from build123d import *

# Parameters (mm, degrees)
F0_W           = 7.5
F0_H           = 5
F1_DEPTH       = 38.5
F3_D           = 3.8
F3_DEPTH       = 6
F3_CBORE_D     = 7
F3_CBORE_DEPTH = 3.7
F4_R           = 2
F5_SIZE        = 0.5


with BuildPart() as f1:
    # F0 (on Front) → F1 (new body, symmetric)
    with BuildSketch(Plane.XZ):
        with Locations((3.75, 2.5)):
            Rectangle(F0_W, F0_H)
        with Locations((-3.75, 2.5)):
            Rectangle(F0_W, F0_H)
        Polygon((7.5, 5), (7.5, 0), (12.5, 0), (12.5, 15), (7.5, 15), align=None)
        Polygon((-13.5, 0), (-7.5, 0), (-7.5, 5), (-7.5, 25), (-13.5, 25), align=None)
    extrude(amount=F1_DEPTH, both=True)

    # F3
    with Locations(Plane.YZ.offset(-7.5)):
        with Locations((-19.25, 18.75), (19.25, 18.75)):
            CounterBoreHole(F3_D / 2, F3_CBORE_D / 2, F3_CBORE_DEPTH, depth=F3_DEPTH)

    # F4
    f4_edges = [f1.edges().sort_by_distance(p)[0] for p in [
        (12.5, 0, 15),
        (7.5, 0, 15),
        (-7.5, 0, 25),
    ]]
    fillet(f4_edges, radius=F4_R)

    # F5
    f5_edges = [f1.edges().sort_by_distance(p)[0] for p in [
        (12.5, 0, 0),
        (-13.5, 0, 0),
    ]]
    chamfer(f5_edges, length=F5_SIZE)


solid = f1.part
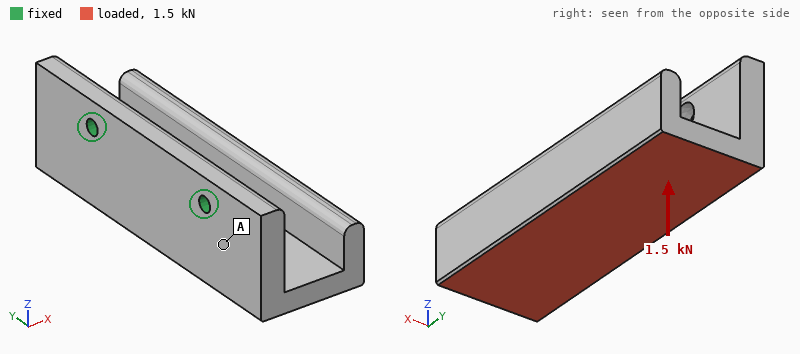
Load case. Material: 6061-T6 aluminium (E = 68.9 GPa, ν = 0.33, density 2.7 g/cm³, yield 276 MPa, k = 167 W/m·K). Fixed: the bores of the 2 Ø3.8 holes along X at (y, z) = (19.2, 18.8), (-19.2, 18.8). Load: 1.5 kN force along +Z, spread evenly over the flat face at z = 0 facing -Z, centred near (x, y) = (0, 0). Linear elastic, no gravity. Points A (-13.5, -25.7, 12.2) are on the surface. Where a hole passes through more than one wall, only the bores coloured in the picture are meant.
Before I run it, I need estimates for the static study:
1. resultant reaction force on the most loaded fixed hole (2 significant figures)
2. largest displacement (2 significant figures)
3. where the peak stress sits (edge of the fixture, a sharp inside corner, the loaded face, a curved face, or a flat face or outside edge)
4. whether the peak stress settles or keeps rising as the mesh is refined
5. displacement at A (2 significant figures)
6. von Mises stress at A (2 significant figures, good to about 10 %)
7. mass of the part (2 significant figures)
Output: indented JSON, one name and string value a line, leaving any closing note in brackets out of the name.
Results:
{
  "resultant reaction force on the most loaded fixed hole": "750 N",
  "largest displacement": "0.29 mm",
  "where the peak stress sits": "edge of the fixture",
  "whether the peak stress settles or keeps rising as the mesh is refined": "keeps rising",
  "displacement at A": "0.044 mm",
  "von Mises stress at A": "36 MPa",
  "mass of the part": "61 g"
}
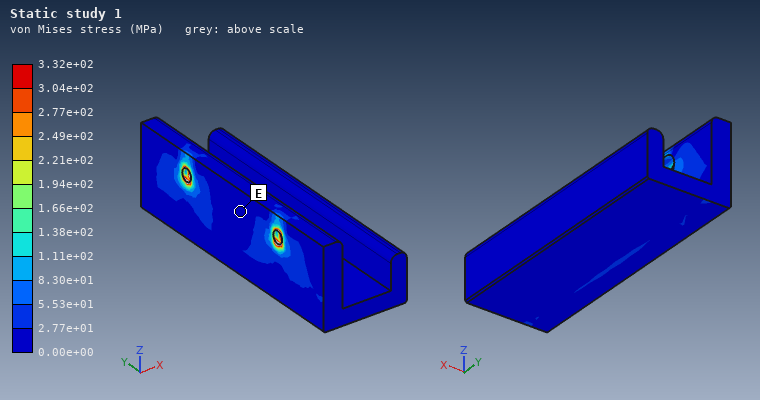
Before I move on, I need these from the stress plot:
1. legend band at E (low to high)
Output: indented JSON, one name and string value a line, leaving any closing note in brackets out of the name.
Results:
{
  "legend band at E": "0.00e+00 to 2.77e+01 MPa"
}
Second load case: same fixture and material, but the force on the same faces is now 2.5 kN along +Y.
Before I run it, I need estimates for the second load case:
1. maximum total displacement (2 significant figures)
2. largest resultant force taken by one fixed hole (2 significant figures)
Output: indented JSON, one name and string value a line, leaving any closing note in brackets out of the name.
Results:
{
  "maximum total displacement": "72 µm",
  "largest resultant force taken by one fixed hole": "1.9 kN"
}
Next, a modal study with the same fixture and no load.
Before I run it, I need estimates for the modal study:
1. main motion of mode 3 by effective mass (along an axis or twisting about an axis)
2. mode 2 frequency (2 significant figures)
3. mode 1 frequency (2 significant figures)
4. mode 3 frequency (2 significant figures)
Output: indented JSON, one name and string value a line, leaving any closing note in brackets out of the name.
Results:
{
  "main motion of mode 3 by effective mass": "along X",
  "mode 2 frequency": "3100 Hz",
  "mode 1 frequency": "1600 Hz",
  "mode 3 frequency": "5500 Hz"
}
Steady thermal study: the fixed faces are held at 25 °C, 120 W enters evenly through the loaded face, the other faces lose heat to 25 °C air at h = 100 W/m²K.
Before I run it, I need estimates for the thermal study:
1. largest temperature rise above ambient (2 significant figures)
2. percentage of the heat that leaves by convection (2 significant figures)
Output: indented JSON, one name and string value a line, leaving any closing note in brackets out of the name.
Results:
{
  "largest temperature rise above ambient": "53 K",
  "percentage of the heat that leaves by convection": "25 %"
}
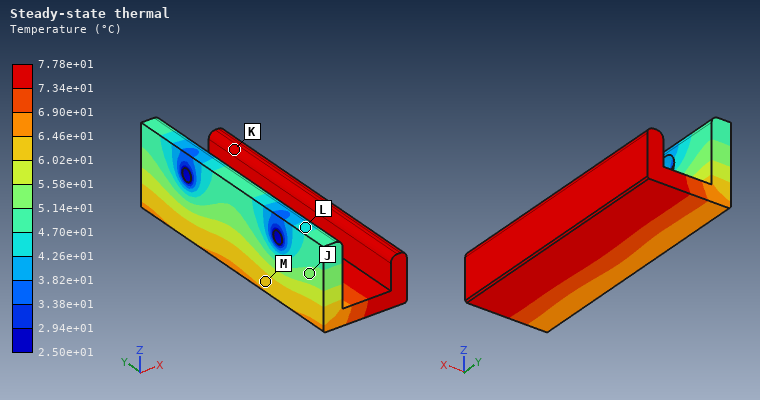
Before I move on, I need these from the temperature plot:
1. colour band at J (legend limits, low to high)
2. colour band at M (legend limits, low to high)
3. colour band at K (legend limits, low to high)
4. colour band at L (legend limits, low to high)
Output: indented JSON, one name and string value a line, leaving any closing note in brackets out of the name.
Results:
{
  "colour band at J": "5.14e+01 to 5.58e+01 °C",
  "colour band at M": "6.02e+01 to 6.46e+01 °C",
  "colour band at K": "7.34e+01 to 7.78e+01 °C",
  "colour band at L": "4.26e+01 to 4.70e+01 °C"
}
